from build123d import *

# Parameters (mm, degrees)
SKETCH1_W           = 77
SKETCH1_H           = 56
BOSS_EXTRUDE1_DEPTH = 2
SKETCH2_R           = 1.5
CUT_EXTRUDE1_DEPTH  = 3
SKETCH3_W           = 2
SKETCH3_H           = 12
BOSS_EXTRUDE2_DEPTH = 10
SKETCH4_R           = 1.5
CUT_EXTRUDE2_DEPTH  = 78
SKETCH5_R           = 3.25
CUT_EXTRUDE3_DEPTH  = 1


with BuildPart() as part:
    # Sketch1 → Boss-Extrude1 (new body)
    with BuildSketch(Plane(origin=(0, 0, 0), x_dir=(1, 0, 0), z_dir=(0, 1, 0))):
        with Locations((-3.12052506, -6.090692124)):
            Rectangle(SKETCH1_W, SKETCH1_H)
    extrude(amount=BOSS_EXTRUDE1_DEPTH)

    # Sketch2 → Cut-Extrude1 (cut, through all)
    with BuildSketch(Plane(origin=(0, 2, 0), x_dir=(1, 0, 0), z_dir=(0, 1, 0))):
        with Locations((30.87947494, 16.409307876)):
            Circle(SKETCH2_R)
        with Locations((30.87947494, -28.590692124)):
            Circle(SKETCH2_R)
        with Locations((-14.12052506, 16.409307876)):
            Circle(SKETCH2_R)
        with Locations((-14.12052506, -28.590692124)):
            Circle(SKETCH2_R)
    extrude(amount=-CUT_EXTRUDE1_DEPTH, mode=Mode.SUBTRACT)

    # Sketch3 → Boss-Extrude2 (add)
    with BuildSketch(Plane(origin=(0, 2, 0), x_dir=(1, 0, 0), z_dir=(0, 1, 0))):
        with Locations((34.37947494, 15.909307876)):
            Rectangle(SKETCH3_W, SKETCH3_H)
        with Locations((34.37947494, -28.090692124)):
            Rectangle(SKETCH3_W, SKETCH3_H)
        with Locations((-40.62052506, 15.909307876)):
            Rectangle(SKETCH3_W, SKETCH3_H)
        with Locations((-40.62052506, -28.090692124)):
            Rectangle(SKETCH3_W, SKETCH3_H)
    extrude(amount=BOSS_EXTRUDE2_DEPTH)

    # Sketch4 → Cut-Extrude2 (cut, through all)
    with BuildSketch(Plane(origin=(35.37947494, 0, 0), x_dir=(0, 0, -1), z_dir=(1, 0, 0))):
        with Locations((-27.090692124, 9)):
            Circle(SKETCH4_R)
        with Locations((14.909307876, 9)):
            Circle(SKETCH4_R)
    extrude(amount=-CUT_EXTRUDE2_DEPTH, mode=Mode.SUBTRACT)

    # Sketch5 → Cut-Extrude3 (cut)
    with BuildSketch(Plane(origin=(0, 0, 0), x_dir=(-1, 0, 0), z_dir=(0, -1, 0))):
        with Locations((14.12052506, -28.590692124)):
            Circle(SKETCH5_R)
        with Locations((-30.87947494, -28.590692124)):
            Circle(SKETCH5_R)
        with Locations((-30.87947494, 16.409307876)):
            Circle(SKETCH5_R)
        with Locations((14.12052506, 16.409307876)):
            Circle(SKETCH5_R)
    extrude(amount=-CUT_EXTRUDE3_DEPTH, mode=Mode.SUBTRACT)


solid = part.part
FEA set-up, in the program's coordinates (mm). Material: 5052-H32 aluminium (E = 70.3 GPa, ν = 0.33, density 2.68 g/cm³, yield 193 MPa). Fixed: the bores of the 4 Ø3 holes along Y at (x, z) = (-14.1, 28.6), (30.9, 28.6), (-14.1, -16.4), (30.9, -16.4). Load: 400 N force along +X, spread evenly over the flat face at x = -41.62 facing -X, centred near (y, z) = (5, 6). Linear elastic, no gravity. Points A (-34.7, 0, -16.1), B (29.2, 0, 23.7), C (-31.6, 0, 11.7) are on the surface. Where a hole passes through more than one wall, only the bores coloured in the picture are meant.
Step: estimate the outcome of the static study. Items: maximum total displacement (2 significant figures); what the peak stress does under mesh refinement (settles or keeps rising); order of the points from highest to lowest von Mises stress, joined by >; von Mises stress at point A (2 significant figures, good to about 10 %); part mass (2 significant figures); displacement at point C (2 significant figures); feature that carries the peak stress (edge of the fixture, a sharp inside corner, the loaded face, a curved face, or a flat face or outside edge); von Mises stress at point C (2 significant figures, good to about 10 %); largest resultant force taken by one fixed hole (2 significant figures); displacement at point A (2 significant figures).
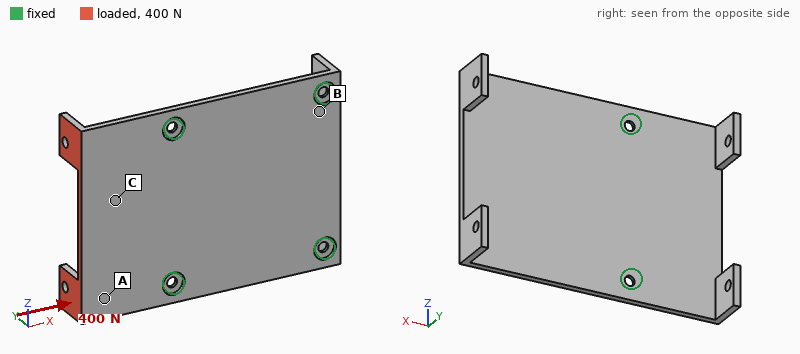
0.42 mm
keeps rising
A > C > B
49 MPa
25 g
0.16 mm
edge of the fixture
29 MPa
240 N
0.19 mm
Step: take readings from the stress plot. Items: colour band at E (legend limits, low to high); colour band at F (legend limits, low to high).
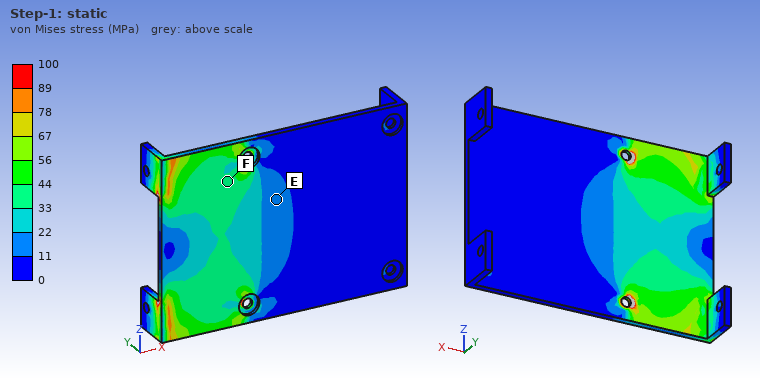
11 to 22 MPa
33 to 44 MPa
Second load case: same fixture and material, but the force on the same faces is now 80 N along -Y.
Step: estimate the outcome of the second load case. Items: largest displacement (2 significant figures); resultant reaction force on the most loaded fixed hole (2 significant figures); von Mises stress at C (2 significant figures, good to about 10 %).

0.40 mm
150 N
21 MPa
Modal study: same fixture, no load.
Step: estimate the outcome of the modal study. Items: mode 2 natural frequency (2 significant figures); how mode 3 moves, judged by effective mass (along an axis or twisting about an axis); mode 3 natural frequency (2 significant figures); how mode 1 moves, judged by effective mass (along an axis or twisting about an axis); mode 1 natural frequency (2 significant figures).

2100 Hz
along Y
3100 Hz
along Y
1300 Hz
